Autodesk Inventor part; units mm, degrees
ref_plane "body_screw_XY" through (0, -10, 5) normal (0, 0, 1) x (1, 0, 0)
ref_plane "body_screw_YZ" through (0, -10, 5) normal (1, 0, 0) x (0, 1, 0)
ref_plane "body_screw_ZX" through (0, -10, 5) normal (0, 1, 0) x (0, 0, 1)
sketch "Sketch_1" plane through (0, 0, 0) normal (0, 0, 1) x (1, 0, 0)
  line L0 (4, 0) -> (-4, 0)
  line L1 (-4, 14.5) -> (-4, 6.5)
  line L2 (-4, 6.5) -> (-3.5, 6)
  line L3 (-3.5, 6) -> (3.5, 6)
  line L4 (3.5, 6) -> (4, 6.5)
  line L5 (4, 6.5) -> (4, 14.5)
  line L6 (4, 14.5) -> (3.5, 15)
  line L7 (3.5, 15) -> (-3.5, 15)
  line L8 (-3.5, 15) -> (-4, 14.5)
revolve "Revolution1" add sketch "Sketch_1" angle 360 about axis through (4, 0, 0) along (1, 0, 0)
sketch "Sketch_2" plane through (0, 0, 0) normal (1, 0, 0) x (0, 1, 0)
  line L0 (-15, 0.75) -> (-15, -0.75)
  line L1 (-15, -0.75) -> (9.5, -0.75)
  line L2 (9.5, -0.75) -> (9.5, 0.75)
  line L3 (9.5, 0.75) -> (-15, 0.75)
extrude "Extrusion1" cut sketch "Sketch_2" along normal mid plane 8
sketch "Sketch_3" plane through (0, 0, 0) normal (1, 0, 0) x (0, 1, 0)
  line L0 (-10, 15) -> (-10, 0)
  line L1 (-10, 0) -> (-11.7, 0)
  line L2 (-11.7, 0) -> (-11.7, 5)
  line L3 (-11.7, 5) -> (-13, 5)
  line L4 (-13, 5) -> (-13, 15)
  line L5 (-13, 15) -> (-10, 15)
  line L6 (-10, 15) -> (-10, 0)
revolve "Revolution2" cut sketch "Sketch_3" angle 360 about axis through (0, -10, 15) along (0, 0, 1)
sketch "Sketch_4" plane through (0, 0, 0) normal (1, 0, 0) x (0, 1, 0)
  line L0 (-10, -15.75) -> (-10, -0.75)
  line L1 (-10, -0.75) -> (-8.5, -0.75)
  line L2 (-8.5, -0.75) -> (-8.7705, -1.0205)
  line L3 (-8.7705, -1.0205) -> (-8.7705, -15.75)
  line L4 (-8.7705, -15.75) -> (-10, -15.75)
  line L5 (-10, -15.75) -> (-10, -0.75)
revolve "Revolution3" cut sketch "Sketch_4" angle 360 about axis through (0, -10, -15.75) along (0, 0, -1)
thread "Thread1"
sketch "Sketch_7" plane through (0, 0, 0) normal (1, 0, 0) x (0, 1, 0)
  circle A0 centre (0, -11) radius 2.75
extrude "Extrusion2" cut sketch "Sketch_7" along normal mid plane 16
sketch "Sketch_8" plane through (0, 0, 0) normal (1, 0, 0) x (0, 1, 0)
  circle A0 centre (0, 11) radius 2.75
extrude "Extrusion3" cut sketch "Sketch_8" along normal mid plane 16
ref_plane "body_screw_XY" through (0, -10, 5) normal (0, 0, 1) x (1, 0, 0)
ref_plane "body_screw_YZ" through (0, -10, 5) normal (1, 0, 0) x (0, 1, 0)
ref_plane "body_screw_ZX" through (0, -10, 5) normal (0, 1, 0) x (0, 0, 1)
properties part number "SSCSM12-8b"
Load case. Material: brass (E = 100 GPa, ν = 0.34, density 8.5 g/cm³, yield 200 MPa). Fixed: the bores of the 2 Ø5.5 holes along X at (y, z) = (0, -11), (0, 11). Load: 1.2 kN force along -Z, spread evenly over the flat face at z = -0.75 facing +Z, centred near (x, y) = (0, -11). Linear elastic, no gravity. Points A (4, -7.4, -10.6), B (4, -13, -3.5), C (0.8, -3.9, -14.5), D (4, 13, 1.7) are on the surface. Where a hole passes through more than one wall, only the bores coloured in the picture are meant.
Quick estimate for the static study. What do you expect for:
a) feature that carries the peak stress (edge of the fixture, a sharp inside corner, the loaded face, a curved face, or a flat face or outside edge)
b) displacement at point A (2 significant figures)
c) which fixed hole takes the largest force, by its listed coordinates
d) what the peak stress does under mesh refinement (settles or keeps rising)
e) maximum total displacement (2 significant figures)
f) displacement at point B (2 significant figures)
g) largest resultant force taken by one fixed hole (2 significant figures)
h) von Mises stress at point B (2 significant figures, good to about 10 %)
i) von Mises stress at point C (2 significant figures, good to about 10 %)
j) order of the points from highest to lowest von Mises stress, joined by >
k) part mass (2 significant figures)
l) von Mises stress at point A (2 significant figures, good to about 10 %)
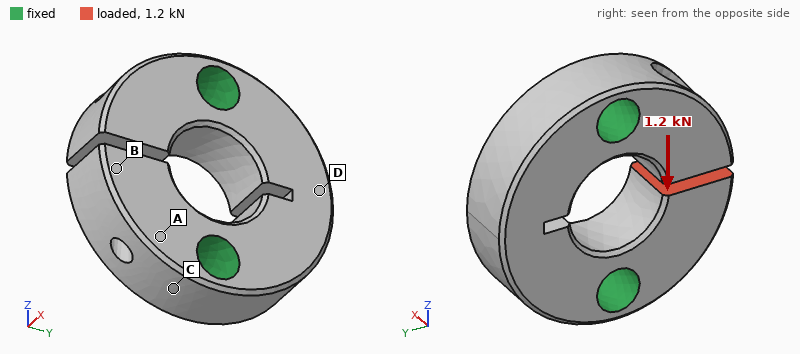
edge of the fixture
6.9 µm
(0, -11)
keeps rising
28 µm
21 µm
1.2 kN
23 MPa
62 MPa
C > A > B > D
33 g
46 MPa
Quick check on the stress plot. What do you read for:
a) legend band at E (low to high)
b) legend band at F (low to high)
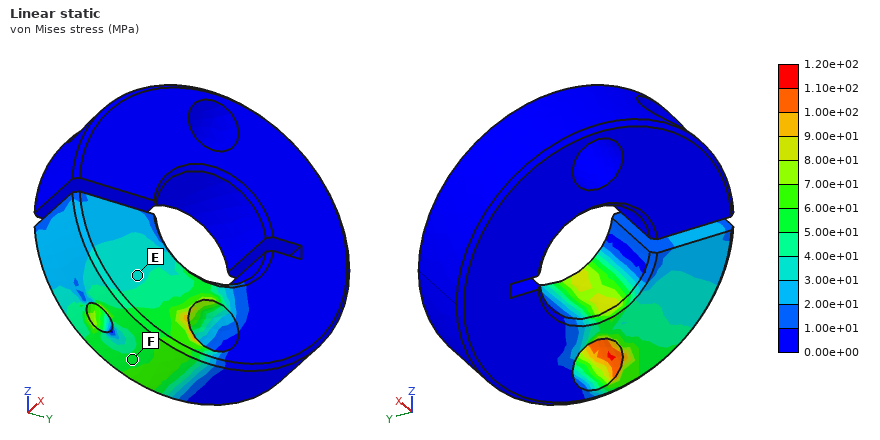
3.00e+01 to 4.00e+01 MPa
5.00e+01 to 6.00e+01 MPa
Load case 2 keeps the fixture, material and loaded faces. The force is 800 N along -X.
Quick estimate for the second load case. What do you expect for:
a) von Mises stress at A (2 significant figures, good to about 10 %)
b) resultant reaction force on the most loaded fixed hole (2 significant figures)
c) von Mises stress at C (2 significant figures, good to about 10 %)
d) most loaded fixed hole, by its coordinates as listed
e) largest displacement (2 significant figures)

58 MPa
800 N
40 MPa
(0, -11)
29 µm
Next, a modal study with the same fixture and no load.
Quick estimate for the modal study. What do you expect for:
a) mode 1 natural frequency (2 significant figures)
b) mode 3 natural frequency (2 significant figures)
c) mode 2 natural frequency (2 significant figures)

17 kHz
18 kHz
18 kHz
